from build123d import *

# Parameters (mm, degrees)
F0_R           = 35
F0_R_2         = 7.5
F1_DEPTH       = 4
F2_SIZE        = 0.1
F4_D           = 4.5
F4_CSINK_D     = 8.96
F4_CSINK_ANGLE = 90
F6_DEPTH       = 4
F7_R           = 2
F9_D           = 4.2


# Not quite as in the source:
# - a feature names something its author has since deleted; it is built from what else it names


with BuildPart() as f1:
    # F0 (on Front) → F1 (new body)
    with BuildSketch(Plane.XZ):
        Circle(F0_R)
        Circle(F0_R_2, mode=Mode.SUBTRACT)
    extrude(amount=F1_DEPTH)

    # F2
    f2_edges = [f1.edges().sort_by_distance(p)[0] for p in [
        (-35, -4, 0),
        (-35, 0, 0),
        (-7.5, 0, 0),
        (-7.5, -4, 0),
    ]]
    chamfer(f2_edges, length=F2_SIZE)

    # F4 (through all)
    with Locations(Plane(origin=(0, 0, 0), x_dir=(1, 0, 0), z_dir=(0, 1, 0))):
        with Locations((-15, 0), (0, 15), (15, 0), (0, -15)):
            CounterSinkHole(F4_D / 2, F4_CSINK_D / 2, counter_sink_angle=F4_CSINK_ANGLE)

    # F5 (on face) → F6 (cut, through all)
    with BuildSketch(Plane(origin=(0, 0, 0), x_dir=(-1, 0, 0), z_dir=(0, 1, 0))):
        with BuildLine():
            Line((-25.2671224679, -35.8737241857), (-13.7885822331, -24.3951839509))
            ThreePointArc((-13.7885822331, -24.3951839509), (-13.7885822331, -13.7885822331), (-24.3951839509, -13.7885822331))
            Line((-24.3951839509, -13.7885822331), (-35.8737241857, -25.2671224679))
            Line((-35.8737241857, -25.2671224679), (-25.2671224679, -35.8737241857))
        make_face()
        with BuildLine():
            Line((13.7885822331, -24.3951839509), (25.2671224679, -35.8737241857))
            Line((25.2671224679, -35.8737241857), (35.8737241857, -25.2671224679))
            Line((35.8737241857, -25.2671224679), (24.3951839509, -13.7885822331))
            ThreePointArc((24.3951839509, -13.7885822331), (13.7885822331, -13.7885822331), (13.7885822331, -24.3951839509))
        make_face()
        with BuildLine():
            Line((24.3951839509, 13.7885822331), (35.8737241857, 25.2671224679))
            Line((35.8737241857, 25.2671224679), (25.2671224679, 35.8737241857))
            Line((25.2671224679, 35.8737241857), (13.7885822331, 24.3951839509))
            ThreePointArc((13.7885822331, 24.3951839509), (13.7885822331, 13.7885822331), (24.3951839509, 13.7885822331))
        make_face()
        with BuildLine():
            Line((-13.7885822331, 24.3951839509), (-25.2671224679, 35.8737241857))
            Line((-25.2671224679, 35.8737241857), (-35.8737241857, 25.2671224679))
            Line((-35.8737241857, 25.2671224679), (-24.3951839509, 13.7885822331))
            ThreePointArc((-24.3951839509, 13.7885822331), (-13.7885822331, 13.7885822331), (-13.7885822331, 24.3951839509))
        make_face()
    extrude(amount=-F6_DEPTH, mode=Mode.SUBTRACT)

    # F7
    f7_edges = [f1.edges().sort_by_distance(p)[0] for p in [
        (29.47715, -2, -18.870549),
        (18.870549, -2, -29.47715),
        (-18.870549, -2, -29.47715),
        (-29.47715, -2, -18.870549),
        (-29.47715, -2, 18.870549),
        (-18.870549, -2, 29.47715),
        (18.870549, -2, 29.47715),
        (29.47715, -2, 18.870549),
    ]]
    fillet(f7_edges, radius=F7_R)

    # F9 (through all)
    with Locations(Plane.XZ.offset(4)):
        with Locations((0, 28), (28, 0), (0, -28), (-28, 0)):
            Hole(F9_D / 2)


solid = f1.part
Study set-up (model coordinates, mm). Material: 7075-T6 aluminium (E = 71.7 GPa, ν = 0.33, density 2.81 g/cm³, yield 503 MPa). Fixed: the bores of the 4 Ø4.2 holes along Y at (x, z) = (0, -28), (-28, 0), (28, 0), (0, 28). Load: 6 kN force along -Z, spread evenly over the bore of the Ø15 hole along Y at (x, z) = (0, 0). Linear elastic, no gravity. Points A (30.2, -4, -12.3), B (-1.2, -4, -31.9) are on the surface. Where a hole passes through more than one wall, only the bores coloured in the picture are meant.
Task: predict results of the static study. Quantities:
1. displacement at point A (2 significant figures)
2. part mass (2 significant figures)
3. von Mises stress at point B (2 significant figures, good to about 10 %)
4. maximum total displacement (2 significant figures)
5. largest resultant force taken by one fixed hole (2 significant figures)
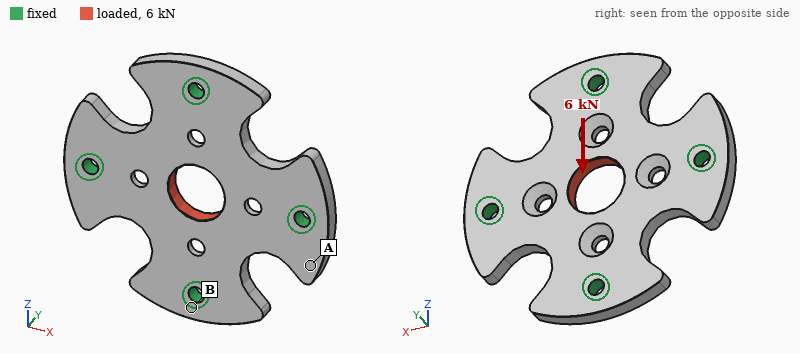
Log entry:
5.6 µm
30 g
25 MPa
16 µm
2.5 kN
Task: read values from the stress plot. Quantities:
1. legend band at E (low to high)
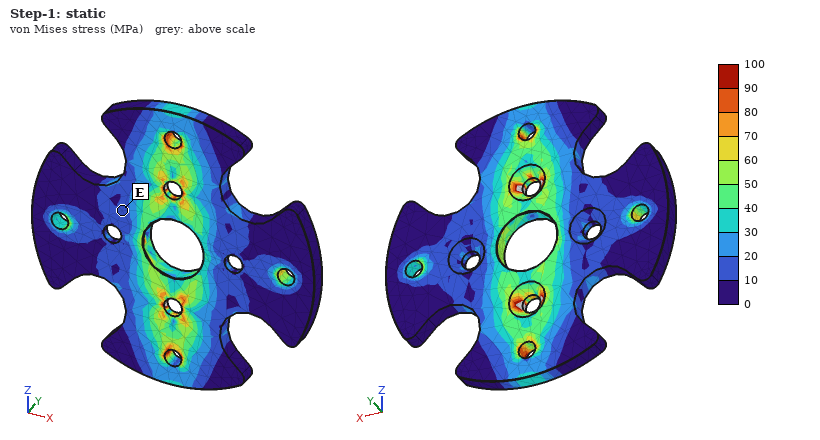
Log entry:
10 to 20 MPa
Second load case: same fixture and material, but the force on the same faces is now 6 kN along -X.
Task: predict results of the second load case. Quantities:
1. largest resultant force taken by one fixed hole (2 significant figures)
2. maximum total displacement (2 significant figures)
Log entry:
2.5 kN
16 µm
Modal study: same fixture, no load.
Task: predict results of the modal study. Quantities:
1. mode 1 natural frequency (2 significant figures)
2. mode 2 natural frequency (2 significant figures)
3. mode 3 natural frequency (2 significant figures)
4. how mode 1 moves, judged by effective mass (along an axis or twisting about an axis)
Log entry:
9900 Hz
14 kHz
14 kHz
along Y
